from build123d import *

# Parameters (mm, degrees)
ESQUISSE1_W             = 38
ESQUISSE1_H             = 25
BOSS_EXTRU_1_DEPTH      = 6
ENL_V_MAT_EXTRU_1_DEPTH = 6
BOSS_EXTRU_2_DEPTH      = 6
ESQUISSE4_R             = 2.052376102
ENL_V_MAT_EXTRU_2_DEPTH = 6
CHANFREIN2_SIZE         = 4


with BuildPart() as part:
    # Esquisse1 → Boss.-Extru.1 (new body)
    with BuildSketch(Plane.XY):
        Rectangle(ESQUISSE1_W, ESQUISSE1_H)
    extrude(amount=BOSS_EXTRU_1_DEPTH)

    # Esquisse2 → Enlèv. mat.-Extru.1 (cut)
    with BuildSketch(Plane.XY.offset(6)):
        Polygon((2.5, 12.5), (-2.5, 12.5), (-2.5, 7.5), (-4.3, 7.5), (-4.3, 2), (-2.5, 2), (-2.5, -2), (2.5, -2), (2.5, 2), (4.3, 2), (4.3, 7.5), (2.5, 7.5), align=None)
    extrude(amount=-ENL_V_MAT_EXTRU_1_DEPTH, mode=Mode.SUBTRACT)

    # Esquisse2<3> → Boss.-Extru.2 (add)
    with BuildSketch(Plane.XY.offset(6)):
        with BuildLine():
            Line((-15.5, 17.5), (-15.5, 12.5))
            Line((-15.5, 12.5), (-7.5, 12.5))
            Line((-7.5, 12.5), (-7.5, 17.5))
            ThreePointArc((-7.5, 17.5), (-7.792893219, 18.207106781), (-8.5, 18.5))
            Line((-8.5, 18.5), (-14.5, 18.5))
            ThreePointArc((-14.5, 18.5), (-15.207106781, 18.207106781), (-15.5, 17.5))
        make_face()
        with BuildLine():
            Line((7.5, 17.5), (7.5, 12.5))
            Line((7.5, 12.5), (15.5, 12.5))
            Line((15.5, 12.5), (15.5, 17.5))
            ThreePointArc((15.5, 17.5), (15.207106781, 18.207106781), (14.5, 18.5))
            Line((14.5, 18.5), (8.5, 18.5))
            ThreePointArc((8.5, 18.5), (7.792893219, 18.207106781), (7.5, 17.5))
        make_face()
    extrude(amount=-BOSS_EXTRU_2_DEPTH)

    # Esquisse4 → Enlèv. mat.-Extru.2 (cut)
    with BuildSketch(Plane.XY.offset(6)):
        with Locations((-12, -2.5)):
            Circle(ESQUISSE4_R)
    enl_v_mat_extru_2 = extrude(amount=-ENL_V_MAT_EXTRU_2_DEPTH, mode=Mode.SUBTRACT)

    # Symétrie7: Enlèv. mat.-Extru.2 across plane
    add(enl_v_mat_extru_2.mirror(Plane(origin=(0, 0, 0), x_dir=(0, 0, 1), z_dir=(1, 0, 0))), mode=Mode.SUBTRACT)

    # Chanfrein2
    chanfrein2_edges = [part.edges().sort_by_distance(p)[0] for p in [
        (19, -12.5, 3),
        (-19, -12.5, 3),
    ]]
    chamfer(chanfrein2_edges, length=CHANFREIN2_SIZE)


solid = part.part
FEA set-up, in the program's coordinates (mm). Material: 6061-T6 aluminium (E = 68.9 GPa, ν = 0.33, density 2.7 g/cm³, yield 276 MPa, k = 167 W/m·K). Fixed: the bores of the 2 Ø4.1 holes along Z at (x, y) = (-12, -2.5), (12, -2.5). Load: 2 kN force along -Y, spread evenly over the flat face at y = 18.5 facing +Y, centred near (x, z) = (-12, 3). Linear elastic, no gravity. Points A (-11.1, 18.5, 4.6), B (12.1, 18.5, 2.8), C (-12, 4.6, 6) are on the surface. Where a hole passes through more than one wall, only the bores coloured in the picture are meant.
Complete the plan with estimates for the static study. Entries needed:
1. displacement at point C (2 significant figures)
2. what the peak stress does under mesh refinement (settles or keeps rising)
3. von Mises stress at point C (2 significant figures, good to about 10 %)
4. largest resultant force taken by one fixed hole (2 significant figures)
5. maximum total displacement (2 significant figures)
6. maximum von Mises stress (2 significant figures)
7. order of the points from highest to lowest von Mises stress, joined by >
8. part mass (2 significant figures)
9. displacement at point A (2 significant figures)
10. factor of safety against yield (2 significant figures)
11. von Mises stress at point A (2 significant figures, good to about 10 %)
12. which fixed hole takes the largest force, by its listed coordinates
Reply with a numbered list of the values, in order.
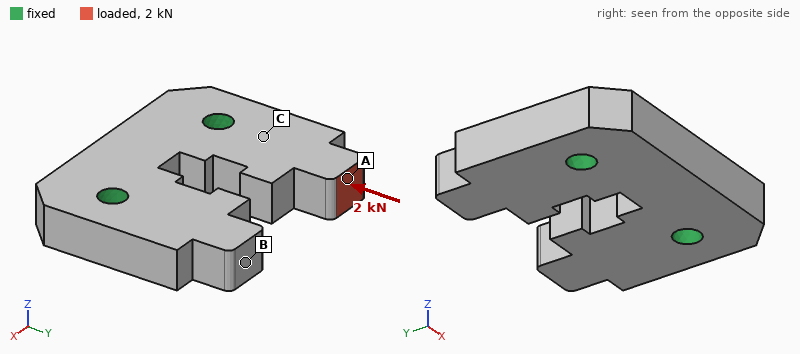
1. 2.7 µm
2. settles
3. 34 MPa
4. 1.9 kN
5. 11 µm
6. 65 MPa
7. A > C > B
8. 15 g
9. 11 µm
10. 4.3
11. 47 MPa
12. (-12, -2.5)
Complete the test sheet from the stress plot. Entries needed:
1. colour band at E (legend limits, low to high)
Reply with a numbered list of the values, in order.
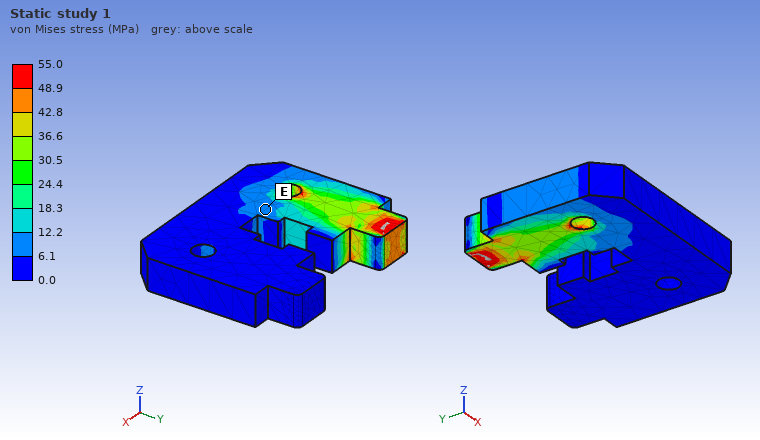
1. 6.1 to 12.2 MPa
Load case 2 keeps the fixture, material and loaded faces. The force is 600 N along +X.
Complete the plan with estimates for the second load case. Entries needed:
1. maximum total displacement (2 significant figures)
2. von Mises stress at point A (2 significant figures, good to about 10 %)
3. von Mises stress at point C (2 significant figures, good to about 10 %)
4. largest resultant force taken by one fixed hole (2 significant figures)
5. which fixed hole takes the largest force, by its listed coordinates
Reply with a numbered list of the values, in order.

1. 38 µm
2. 30 MPa
3. 16 MPa
4. 930 N
5. (-12, -2.5)
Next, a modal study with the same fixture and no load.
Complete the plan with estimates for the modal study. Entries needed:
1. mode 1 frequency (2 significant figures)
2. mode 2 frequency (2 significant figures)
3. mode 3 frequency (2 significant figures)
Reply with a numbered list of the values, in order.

1. 13 kHz
2. 13 kHz
3. 19 kHz
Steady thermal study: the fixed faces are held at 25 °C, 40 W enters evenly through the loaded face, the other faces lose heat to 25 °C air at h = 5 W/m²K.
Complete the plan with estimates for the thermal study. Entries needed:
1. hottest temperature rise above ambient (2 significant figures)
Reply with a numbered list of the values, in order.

1. 76 K
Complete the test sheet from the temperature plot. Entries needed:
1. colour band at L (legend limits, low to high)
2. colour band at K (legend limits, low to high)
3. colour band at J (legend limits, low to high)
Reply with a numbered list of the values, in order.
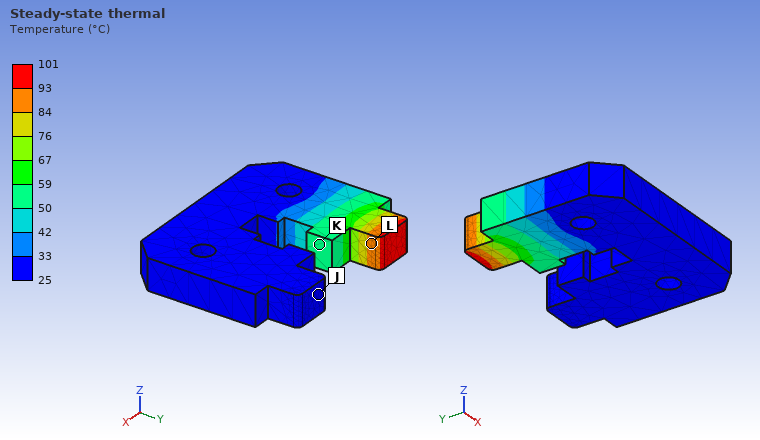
1. 84 to 93 °C
2. 50 to 59 °C
3. 25 to 33 °C
